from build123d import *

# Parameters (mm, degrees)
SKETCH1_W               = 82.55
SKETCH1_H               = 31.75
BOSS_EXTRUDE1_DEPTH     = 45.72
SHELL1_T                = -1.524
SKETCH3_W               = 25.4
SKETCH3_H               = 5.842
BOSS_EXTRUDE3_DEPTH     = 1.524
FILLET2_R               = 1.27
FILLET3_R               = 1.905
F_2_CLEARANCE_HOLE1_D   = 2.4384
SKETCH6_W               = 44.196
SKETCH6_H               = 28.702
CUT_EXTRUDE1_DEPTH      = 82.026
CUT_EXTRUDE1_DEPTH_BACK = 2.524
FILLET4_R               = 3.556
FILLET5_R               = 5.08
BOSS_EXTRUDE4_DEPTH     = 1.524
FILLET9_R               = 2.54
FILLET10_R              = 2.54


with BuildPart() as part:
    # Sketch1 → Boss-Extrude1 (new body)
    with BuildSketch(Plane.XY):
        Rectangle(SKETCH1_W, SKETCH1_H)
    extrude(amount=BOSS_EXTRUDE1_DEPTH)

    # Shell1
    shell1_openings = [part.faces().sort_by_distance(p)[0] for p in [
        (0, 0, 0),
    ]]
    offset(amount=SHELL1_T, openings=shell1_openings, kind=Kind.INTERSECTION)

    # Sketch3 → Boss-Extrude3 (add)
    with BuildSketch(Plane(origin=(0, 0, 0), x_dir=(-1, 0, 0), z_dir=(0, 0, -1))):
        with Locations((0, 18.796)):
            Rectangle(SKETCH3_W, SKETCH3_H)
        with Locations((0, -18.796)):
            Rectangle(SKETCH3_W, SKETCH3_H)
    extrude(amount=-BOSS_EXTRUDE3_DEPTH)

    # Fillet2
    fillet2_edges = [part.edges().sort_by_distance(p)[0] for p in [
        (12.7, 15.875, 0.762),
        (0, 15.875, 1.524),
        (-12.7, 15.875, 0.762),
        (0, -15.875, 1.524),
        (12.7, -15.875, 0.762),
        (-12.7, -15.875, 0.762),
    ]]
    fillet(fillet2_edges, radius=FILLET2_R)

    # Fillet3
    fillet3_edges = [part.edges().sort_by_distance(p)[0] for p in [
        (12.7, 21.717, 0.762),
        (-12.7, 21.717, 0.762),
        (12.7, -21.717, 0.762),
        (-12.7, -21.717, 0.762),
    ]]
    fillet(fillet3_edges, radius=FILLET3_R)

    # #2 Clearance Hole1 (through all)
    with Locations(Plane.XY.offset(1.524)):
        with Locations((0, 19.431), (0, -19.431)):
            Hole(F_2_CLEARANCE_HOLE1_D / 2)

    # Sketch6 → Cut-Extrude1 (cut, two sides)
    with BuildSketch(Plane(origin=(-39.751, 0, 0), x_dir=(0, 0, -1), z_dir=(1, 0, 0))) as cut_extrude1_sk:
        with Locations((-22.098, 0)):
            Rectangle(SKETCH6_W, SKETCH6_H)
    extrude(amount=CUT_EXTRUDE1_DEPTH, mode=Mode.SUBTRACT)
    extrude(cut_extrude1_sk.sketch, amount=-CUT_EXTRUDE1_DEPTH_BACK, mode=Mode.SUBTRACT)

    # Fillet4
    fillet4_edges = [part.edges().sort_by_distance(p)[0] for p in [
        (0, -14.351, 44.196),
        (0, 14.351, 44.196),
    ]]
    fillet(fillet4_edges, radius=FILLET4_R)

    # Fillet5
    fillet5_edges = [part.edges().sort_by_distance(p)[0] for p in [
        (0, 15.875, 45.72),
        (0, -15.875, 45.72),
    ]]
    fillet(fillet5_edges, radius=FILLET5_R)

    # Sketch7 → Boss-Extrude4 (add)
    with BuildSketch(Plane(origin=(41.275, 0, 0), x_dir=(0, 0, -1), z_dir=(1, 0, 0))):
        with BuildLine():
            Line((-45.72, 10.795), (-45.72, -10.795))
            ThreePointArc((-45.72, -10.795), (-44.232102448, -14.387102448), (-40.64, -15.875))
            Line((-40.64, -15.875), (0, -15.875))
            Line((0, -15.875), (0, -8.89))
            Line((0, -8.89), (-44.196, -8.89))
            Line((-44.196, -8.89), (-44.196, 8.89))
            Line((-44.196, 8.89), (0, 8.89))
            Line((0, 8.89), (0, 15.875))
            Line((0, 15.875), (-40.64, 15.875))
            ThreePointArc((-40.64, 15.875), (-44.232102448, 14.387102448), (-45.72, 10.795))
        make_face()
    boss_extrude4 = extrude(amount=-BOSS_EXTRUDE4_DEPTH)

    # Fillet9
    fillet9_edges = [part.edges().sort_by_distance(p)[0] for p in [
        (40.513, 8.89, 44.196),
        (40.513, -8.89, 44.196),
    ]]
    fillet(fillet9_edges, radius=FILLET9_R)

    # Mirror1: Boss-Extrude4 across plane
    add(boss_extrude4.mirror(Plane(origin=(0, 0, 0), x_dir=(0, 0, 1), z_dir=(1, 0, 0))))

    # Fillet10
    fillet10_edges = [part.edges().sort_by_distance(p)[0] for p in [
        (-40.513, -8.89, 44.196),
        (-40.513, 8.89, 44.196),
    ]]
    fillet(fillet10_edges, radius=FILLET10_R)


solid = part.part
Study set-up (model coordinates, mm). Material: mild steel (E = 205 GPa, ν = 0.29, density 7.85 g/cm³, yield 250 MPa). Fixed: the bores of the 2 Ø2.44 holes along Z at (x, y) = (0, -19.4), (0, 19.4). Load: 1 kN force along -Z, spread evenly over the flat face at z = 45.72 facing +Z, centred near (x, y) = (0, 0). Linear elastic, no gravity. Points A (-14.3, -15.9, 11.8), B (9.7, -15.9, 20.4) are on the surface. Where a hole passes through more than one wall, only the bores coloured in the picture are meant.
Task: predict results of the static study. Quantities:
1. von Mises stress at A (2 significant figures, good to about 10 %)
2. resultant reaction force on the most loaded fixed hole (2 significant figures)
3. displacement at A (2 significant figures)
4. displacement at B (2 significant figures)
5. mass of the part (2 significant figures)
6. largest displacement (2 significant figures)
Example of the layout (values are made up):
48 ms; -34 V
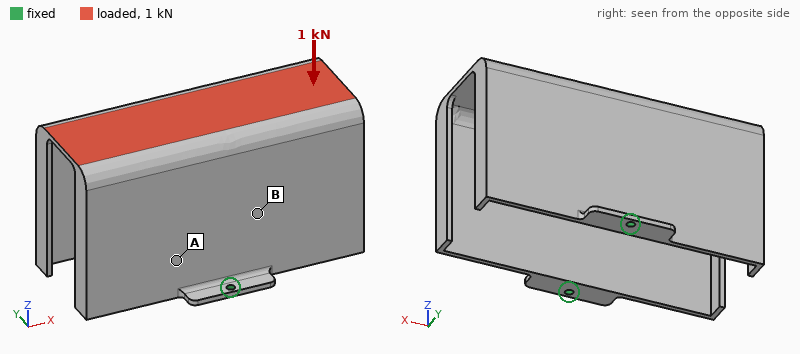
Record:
16 MPa; 510 N; 13 µm; 16 µm; 130 g; 71 µm
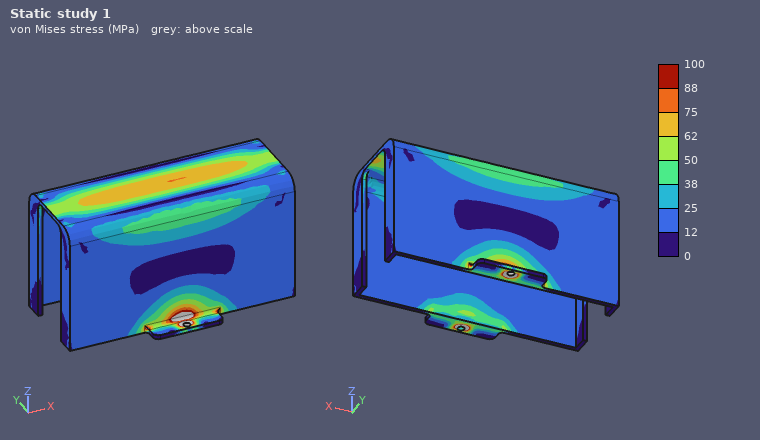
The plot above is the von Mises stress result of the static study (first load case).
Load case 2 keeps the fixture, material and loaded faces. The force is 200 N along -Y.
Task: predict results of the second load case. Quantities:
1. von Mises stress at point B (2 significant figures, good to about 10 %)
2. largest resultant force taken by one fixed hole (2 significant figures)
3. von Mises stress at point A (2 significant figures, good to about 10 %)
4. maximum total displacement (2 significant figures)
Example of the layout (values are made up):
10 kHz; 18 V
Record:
16 MPa; 240 N; 25 MPa; 0.22 mm
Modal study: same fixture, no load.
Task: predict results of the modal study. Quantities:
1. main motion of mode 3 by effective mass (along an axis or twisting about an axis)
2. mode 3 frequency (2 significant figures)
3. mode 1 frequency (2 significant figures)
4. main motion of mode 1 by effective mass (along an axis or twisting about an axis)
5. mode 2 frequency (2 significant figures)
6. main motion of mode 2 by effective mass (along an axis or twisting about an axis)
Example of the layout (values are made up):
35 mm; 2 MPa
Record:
twisting about Z; 640 Hz; 330 Hz; along X; 550 Hz; along Y
